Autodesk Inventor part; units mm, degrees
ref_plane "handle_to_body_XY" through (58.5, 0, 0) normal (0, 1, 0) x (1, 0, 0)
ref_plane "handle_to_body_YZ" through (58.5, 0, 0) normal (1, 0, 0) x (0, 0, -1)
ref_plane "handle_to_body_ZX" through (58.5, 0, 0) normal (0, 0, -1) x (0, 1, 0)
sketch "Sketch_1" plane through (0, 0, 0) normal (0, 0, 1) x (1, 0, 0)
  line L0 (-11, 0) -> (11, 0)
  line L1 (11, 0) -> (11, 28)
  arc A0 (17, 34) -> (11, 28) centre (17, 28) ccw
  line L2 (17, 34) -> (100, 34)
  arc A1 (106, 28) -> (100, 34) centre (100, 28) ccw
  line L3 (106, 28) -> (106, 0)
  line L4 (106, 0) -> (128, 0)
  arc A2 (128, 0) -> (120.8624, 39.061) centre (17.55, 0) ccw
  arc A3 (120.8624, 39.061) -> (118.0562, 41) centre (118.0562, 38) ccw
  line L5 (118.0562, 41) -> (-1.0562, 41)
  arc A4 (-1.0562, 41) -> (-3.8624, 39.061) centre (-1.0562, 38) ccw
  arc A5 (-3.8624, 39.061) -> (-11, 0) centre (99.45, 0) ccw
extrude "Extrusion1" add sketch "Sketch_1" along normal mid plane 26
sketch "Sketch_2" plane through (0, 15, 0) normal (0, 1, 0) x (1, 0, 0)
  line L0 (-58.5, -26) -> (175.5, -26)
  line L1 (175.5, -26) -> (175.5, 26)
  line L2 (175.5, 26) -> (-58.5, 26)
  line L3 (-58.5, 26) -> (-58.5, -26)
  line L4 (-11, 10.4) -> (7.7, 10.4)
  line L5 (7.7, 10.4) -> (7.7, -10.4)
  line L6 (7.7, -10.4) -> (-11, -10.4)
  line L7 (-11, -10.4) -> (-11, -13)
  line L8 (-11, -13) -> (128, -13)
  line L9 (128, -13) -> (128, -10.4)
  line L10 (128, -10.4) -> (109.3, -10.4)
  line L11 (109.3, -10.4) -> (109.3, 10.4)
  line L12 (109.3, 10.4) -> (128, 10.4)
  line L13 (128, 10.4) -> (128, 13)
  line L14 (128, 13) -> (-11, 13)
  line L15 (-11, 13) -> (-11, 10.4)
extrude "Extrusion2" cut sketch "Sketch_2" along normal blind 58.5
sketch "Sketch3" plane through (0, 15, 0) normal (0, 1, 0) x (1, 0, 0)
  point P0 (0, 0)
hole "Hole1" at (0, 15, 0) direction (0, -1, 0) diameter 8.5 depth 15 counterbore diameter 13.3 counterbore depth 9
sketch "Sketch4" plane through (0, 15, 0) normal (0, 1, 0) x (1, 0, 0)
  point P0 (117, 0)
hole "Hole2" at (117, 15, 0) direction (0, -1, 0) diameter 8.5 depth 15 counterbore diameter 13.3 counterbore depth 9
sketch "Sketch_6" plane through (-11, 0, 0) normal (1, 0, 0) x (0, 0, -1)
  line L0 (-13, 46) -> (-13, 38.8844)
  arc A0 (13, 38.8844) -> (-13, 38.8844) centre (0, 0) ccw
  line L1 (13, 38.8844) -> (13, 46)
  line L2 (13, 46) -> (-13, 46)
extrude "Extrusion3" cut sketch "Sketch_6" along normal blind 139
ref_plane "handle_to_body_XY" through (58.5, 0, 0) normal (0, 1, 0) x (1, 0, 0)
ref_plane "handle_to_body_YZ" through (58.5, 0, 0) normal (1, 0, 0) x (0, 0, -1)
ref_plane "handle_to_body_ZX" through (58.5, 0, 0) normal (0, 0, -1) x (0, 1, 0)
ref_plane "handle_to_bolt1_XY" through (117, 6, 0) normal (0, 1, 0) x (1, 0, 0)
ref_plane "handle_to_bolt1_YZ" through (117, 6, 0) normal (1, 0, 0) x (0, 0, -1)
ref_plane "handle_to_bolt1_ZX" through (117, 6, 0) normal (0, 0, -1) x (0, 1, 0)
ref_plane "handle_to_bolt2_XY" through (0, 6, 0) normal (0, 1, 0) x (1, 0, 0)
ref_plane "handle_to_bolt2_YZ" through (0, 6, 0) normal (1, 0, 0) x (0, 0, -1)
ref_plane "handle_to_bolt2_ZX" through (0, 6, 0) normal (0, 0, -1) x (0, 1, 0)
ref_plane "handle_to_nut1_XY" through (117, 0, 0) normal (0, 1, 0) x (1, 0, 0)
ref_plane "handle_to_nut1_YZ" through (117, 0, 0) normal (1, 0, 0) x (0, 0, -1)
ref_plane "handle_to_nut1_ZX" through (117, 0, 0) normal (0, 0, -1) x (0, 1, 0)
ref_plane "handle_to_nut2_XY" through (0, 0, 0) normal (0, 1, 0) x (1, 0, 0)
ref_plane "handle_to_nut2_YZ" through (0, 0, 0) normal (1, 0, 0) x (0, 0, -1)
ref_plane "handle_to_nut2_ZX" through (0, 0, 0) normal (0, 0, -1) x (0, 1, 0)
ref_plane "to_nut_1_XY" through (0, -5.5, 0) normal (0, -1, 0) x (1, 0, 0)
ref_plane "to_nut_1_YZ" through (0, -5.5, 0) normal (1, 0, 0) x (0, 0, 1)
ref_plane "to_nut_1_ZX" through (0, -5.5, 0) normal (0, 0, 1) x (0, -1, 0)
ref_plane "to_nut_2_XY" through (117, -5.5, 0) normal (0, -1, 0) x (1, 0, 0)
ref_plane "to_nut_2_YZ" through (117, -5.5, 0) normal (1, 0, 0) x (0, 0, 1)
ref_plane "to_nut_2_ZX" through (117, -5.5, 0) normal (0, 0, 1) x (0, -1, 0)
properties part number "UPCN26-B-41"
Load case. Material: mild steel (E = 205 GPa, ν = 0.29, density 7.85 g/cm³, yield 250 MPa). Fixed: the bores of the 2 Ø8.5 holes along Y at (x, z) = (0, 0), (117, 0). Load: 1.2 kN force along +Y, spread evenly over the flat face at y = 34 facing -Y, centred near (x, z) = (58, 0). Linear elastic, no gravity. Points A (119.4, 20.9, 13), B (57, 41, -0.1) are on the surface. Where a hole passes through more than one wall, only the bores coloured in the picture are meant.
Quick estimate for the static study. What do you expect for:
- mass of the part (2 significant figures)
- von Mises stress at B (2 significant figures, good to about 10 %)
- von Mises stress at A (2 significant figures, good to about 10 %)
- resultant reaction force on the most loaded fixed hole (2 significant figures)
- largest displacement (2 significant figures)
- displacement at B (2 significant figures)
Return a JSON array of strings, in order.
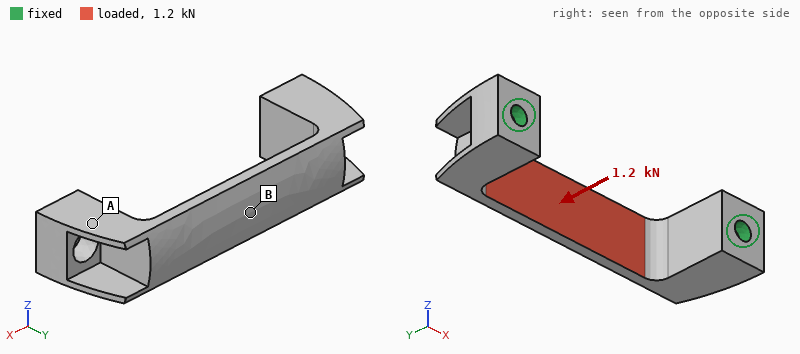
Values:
["300 g", "46 MPa", "8.1 MPa", "790 N", "41 µm", "40 µm"]
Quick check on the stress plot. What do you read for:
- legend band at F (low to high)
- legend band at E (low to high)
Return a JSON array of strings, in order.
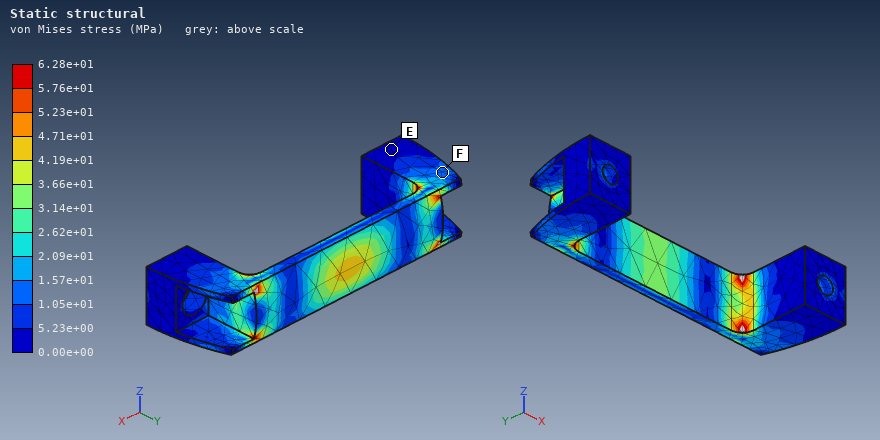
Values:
["1.05e+01 to 1.57e+01 MPa", "0.00e+00 to 5.23e+00 MPa"]
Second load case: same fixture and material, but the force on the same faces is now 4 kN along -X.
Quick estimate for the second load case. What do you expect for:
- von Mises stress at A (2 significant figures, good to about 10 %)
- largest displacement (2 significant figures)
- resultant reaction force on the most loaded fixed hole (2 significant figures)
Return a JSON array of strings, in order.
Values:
["36 MPa", "49 µm", "2.0 kN"]
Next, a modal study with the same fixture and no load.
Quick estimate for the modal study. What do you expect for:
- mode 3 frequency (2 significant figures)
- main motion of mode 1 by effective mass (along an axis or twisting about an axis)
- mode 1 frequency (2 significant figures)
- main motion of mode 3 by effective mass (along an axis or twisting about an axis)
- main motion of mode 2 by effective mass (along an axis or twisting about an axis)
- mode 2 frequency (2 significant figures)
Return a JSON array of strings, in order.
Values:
["3700 Hz", "along Y", "3000 Hz", "along X", "along Z", "3200 Hz"]
